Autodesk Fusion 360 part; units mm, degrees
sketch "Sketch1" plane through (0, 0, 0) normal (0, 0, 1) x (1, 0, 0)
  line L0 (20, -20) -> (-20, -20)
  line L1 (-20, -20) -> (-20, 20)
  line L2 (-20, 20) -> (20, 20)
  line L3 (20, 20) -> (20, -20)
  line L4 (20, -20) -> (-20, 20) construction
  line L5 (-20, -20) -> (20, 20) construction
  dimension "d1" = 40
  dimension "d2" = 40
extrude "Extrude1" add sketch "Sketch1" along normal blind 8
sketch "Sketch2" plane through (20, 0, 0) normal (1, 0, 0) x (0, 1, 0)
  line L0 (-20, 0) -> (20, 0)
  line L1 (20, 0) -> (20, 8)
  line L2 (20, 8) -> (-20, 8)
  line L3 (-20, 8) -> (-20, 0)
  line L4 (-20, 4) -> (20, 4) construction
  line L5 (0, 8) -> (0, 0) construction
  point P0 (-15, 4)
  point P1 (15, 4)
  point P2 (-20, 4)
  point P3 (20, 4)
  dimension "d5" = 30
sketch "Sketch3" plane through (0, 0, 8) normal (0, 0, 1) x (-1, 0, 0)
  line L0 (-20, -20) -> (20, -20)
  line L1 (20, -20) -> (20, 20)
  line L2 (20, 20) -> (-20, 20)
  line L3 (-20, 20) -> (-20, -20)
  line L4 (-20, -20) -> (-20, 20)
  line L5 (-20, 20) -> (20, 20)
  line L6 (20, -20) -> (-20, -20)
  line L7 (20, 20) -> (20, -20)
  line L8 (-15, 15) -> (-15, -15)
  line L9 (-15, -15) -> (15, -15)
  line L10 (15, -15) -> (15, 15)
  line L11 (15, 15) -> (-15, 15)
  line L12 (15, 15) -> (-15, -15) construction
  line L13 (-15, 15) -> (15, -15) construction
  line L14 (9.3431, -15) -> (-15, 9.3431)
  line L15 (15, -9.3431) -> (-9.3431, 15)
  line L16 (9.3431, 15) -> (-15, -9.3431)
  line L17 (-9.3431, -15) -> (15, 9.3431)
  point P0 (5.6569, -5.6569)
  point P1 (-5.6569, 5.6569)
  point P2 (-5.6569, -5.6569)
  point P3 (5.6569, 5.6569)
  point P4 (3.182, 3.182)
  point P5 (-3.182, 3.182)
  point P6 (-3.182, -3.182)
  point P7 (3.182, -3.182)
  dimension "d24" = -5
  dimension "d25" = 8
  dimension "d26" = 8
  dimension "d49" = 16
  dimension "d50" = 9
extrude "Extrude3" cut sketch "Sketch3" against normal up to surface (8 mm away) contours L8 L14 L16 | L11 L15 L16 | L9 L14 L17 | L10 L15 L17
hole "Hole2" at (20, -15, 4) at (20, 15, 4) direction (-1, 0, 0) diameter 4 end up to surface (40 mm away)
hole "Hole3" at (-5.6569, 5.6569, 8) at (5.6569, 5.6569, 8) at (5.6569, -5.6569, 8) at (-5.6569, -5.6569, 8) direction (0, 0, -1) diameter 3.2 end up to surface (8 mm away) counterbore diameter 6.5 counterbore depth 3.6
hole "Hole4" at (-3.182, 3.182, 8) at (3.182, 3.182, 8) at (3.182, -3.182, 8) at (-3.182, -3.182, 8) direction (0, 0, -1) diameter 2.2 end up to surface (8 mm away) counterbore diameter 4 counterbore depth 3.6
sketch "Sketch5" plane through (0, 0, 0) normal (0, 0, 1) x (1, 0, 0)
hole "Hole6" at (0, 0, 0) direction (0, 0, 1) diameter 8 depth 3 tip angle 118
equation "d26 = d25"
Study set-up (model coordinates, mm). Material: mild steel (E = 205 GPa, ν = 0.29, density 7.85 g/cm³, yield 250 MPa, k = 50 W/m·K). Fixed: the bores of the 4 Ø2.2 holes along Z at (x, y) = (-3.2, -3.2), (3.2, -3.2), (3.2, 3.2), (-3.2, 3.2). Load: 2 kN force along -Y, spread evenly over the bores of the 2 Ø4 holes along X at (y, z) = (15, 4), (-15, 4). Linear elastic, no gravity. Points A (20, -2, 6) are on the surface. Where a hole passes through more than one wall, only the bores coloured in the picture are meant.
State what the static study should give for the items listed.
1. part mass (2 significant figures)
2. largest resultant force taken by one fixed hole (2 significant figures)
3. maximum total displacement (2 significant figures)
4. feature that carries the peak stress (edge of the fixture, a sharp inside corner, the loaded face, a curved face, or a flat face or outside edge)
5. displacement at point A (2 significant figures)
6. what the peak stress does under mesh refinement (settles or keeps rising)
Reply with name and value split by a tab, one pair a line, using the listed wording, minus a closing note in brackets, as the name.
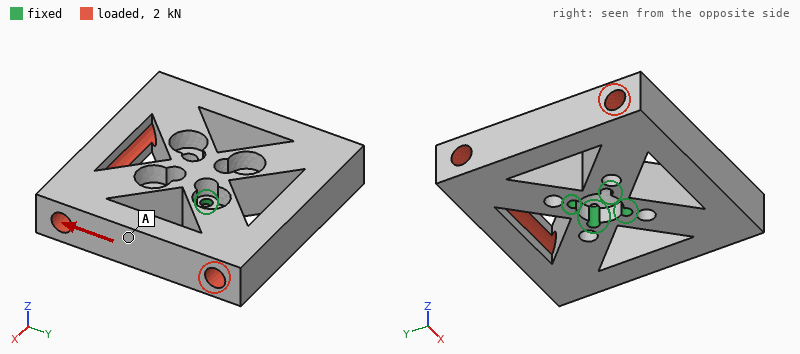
part mass	65 g
largest resultant force taken by one fixed hole	520 N
maximum total displacement	6.6 µm
feature that carries the peak stress	a sharp inside corner
displacement at point A	3.4 µm
what the peak stress does under mesh refinement	keeps rising
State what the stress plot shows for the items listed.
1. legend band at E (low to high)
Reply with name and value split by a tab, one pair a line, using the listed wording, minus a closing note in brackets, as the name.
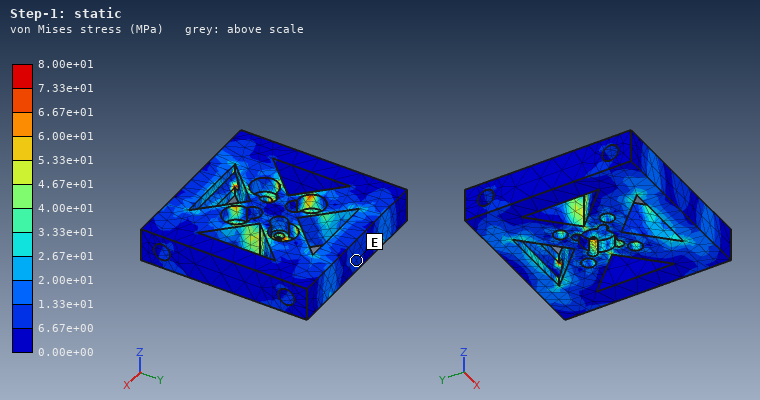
legend band at E	6.67e+00 to 1.33e+01 MPa
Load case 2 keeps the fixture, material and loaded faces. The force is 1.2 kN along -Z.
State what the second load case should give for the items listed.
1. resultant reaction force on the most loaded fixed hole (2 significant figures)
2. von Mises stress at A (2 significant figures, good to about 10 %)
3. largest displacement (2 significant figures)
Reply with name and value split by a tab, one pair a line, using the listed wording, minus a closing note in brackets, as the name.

resultant reaction force on the most loaded fixed hole	390 N
von Mises stress at A	15 MPa
largest displacement	14 µm
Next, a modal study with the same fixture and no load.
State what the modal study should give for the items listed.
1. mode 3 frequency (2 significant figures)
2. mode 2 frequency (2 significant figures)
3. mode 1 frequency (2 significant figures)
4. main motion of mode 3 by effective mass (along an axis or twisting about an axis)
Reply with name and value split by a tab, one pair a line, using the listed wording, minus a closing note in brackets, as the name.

mode 3 frequency	7300 Hz
mode 2 frequency	6300 Hz
mode 1 frequency	6300 Hz
main motion of mode 3 by effective mass	twisting about Z
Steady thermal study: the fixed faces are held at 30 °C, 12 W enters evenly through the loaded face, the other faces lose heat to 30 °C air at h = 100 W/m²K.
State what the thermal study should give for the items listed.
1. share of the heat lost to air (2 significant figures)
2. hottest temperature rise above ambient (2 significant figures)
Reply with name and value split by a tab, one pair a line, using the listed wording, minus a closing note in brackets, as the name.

share of the heat lost to air	45 %
hottest temperature rise above ambient	16 K
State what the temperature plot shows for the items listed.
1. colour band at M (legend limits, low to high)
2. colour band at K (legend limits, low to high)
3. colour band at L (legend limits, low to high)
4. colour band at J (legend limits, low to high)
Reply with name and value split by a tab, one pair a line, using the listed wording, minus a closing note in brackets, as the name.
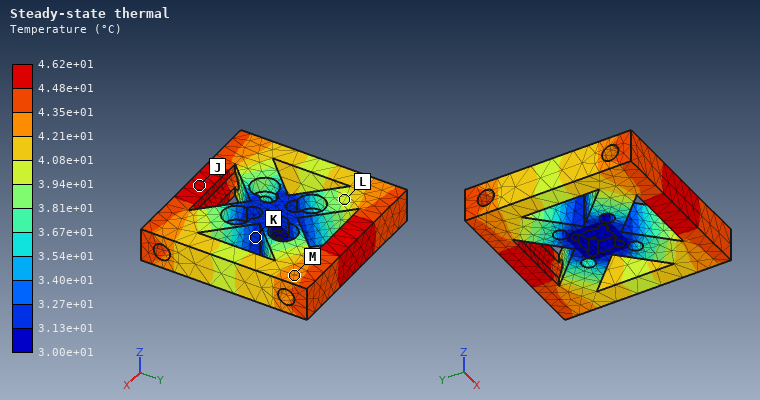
colour band at M	4.21e+01 to 4.35e+01 °C
colour band at K	3.13e+01 to 3.27e+01 °C
colour band at L	3.94e+01 to 4.08e+01 °C
colour band at J	4.48e+01 to 4.62e+01 °C
